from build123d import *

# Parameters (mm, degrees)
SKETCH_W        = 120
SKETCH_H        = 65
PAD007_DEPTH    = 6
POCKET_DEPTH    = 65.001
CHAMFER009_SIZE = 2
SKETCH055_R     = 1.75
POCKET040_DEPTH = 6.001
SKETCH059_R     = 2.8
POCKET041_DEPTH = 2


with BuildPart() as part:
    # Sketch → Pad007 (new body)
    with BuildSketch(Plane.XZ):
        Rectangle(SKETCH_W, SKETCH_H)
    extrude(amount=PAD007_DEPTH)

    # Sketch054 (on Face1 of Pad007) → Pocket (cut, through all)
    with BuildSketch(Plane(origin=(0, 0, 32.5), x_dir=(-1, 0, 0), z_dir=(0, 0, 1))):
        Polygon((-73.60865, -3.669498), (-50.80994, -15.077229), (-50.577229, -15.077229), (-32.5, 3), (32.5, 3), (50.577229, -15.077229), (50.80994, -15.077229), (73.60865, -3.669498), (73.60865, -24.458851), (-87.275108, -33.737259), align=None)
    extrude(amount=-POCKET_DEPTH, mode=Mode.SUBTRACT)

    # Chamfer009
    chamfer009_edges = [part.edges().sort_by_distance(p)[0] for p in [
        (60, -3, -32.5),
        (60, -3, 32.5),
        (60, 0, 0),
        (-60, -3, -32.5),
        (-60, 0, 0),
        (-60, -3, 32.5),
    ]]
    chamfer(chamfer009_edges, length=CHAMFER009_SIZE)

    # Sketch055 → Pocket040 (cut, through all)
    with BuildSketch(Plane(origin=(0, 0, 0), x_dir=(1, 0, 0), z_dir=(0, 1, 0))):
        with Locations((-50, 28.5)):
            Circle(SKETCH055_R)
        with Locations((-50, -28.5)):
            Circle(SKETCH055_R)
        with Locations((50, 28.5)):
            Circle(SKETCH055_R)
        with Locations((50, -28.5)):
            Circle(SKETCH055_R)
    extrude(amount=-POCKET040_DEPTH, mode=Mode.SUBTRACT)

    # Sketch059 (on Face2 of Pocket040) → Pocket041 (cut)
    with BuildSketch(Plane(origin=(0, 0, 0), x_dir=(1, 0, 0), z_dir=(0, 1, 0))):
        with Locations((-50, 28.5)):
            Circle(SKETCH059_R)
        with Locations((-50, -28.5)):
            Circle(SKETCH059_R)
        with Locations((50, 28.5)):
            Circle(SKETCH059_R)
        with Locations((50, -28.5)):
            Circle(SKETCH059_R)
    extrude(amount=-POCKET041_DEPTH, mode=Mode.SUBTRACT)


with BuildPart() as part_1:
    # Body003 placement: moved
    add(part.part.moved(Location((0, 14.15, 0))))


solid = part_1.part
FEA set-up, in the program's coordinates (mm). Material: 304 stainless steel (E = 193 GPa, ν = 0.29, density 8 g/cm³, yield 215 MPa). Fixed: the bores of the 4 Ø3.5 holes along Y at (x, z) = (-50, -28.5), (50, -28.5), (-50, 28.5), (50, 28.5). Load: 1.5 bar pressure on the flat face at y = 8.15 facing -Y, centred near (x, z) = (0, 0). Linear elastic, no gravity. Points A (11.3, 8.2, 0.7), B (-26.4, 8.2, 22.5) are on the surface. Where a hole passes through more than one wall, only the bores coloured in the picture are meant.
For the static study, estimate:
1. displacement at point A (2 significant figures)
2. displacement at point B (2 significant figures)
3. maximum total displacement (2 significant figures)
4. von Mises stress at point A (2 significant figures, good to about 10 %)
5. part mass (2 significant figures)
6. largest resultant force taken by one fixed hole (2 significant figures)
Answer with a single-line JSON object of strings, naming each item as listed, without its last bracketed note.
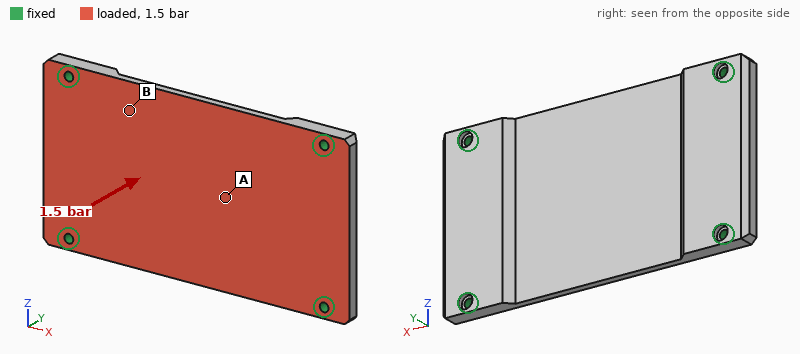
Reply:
{"displacement at point A": "47 µm", "displacement at point B": "24 µm", "maximum total displacement": "52 µm", "von Mises stress at point A": "21 MPa", "part mass": "260 g", "largest resultant force taken by one fixed hole": "440 N"}
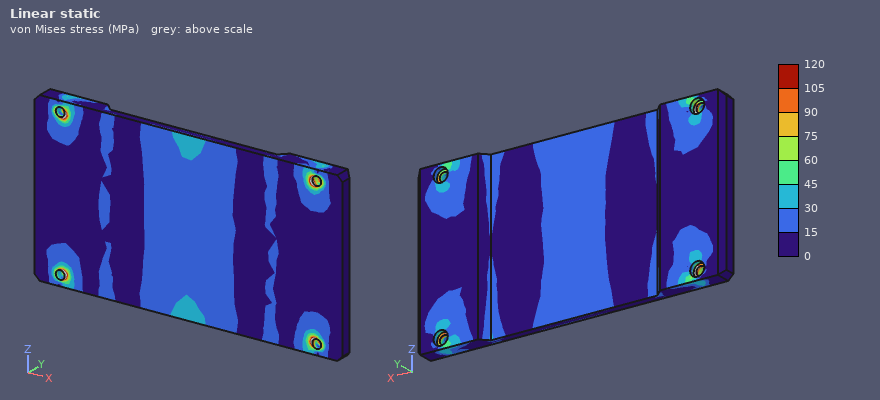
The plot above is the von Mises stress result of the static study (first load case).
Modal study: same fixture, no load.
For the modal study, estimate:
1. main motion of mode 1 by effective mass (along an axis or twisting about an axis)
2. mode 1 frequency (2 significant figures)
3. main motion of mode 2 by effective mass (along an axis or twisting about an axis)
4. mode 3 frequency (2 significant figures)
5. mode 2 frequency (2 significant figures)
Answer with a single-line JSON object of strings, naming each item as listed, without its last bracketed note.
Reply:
{"main motion of mode 1 by effective mass": "along Y", "mode 1 frequency": "2000 Hz", "main motion of mode 2 by effective mass": "twisting about X", "mode 3 frequency": "4200 Hz", "mode 2 frequency": "3200 Hz"}
